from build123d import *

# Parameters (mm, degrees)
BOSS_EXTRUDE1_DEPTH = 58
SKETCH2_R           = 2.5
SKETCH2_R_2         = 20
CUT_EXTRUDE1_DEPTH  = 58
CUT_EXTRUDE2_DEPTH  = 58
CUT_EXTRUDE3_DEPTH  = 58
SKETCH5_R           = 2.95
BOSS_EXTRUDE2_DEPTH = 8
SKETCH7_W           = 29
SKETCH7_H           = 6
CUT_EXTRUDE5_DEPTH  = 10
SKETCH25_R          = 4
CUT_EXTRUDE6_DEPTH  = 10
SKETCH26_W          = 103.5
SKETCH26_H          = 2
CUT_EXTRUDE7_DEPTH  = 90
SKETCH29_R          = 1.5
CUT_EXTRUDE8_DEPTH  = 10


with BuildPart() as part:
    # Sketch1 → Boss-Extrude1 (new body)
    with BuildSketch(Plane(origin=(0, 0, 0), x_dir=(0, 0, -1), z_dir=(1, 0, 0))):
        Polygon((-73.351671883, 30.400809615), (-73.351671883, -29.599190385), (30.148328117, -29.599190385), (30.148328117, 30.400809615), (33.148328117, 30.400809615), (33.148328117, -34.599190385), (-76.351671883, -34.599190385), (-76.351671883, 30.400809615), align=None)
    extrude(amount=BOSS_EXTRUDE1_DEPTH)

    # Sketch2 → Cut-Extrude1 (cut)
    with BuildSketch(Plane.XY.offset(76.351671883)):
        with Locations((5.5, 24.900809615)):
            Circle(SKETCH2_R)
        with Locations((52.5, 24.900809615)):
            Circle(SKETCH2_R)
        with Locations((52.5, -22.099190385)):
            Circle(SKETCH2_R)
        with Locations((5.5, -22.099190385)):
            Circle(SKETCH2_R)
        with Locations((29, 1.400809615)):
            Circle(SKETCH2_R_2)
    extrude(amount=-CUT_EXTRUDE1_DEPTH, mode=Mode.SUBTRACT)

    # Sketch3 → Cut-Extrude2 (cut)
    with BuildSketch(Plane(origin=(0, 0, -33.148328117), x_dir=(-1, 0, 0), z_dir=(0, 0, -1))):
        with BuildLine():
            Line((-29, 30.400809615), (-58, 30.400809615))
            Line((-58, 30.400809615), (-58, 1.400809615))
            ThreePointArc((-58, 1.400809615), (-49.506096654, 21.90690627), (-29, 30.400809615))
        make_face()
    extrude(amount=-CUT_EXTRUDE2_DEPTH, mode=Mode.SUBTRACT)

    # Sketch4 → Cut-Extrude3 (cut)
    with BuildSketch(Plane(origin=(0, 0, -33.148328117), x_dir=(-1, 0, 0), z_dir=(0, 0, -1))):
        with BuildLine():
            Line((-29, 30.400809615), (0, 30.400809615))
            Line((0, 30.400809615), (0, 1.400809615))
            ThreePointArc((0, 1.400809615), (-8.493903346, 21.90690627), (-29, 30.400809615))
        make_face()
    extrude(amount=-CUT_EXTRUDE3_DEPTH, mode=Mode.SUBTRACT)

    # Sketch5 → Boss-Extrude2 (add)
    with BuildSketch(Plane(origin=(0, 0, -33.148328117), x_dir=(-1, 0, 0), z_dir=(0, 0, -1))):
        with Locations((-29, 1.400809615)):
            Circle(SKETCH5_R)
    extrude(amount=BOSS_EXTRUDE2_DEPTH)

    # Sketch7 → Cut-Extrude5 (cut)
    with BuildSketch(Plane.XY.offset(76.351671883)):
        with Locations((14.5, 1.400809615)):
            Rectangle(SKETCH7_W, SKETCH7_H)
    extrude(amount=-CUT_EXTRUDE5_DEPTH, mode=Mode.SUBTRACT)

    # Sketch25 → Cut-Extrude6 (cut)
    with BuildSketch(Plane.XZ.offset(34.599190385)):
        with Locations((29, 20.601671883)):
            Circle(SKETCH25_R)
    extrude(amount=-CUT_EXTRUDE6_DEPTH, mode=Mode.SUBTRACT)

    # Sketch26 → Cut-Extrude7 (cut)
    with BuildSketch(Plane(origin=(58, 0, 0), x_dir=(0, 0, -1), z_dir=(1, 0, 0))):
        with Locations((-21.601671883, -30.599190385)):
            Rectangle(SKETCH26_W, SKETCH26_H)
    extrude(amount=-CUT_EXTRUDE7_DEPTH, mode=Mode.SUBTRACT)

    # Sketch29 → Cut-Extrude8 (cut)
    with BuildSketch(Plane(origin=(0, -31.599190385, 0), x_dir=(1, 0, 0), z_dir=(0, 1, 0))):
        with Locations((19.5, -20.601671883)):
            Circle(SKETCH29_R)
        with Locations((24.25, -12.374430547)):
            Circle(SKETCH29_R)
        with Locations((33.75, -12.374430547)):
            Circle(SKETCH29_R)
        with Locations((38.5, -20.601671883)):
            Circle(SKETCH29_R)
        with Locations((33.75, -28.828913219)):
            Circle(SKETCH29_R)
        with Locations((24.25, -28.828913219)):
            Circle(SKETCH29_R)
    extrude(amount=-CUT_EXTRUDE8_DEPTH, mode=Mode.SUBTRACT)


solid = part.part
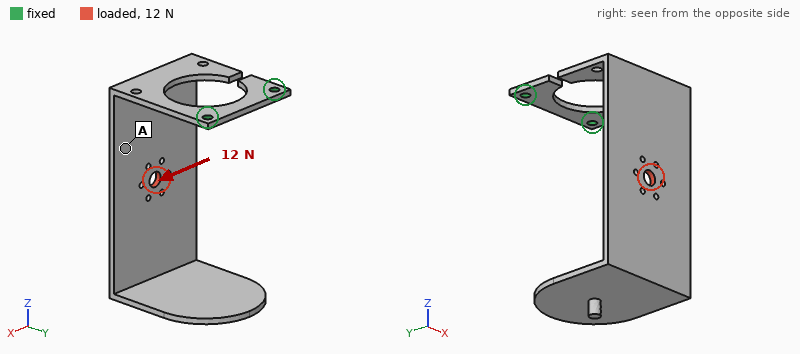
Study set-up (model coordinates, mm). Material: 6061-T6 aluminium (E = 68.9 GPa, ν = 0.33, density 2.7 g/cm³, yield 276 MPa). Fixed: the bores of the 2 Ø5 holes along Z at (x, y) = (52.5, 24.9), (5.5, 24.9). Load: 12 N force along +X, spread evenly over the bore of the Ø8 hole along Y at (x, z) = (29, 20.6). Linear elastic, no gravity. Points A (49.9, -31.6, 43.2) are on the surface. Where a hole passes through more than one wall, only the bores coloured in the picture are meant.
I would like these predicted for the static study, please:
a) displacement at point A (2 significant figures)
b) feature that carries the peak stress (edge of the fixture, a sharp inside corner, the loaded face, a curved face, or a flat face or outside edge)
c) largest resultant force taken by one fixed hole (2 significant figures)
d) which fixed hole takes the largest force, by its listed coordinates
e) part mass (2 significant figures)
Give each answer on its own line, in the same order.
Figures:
0.46 mm
a flat face or outside edge
13 N
(52.5, 24.9)
95 g
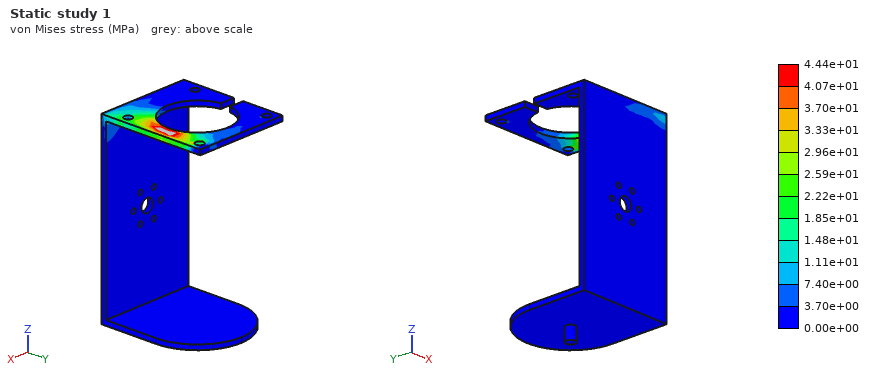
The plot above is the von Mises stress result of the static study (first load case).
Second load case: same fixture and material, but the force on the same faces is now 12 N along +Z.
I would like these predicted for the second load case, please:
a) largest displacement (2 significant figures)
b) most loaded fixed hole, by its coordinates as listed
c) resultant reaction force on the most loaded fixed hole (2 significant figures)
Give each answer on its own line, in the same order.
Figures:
1.5 mm
(52.5, 24.9)
13 N
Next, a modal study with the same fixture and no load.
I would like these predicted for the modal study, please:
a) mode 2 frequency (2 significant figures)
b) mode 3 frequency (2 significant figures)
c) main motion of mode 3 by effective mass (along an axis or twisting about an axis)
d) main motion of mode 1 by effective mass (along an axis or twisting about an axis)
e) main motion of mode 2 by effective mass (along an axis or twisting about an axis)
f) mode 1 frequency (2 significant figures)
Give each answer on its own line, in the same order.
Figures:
47 Hz
170 Hz
along Z
along Y
along X
38 Hz
